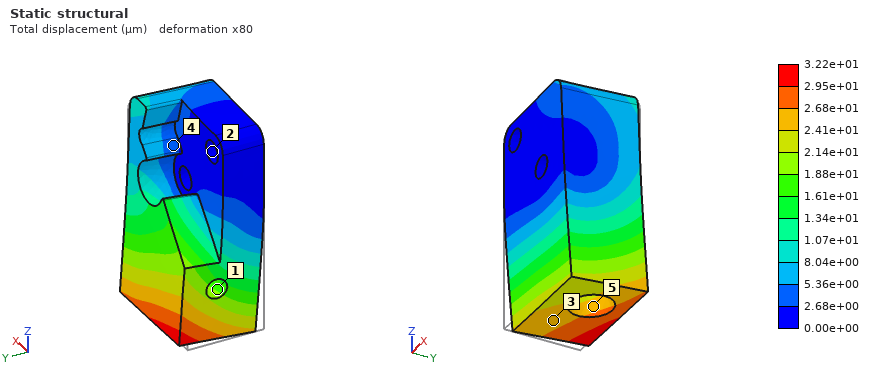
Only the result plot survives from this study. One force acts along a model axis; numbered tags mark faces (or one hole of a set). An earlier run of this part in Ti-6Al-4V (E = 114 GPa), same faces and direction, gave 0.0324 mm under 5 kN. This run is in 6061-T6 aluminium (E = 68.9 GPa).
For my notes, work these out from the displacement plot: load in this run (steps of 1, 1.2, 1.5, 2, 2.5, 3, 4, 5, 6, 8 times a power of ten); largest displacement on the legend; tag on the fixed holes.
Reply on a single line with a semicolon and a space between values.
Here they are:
3 kN; 3.22e+01 µm; 2
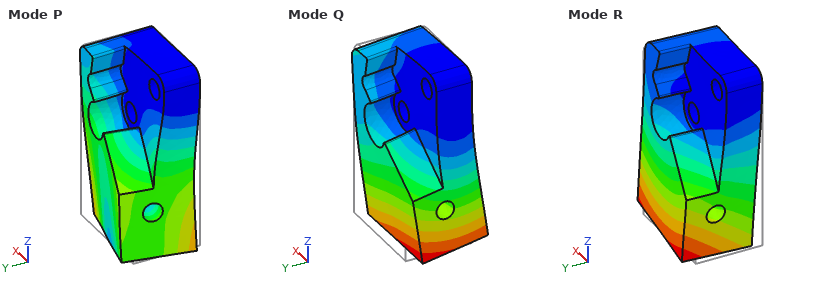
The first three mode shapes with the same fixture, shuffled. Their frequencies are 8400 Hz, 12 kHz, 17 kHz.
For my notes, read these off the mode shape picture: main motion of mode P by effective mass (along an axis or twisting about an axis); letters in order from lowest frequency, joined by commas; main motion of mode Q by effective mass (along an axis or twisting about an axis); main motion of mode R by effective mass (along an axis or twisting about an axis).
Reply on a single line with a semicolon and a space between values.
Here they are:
twisting about Z; Q, R, P; along Y; along X
